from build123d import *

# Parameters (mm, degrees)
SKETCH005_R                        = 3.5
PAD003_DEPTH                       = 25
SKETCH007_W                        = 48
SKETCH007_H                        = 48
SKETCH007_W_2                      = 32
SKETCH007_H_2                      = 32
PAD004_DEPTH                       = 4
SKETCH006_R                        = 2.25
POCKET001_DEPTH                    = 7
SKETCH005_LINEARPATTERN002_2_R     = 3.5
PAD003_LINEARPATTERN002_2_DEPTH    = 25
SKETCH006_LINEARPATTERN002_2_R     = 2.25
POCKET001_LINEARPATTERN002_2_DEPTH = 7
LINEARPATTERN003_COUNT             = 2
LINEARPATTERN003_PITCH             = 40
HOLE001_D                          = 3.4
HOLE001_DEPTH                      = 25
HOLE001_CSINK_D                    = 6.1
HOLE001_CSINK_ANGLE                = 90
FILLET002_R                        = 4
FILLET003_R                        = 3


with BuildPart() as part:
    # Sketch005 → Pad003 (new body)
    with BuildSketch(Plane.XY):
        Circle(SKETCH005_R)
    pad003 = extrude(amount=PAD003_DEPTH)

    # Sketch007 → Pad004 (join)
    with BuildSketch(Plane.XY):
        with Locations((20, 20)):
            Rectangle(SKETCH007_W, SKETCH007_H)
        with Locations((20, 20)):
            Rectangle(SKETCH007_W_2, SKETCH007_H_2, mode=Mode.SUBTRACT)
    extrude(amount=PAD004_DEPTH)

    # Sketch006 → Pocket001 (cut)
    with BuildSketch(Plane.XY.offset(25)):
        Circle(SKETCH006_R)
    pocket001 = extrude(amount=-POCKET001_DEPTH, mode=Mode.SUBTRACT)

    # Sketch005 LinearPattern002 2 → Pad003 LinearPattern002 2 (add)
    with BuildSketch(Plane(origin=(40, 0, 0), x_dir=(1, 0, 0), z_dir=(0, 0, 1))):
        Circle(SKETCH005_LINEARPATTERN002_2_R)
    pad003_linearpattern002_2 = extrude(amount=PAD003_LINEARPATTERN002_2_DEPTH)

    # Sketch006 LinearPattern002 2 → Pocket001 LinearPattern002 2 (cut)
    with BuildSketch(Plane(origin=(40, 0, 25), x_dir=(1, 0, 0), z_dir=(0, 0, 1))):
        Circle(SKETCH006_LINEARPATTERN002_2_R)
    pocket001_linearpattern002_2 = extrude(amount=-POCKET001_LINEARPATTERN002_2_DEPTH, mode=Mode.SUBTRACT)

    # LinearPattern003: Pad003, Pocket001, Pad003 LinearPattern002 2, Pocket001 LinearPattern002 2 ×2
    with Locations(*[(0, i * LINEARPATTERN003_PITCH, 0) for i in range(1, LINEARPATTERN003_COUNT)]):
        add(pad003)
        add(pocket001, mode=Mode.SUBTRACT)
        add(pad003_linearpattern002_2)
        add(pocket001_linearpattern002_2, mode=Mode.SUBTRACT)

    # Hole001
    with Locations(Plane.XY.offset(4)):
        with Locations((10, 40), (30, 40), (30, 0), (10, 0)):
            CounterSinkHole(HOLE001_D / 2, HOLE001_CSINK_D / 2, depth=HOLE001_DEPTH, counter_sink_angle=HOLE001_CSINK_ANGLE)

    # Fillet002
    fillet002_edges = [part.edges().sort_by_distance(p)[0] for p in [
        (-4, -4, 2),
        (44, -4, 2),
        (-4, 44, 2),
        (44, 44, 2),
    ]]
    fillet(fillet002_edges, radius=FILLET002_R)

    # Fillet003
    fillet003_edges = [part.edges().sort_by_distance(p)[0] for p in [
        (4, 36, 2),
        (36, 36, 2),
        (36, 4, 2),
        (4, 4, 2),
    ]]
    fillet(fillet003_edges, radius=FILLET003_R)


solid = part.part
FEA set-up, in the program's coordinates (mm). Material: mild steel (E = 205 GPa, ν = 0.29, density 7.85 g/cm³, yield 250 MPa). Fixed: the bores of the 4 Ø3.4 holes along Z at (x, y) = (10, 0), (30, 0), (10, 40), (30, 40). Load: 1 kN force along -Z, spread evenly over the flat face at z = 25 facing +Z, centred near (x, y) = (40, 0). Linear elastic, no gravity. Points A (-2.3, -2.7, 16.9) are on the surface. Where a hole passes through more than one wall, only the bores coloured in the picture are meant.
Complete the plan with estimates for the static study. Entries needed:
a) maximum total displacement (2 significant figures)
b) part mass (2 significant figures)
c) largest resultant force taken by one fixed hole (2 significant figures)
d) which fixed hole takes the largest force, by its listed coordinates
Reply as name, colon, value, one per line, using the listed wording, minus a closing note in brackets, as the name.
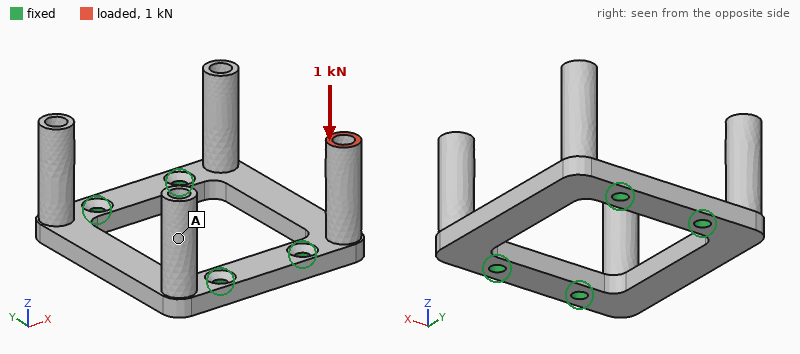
maximum total displacement: 0.13 mm
part mass: 60 g
largest resultant force taken by one fixed hole: 1.0 kN
which fixed hole takes the largest force, by its listed coordinates: (30, 0)
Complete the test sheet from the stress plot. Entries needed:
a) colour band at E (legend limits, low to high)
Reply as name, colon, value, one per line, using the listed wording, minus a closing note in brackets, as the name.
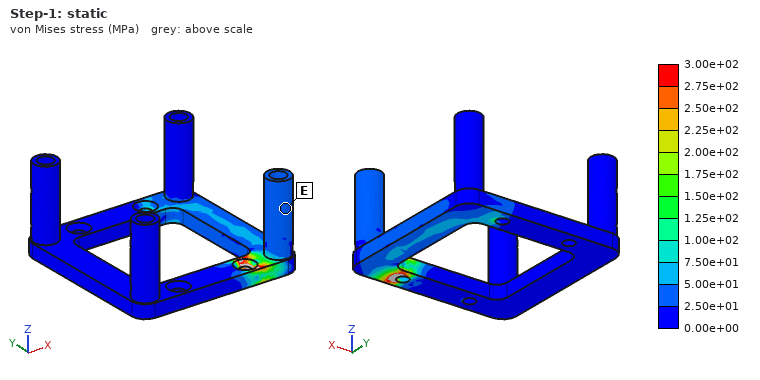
colour band at E: 2.50e+01 to 5.00e+01 MPa
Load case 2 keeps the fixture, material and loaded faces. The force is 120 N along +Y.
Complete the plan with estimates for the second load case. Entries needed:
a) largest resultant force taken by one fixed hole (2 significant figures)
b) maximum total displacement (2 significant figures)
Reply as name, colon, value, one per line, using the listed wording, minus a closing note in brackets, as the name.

largest resultant force taken by one fixed hole: 81 N
maximum total displacement: 52 µm
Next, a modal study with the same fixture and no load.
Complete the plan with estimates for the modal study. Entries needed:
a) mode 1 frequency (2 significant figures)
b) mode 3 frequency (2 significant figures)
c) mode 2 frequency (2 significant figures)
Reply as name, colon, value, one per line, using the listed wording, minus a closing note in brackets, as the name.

mode 1 frequency: 4000 Hz
mode 3 frequency: 5000 Hz
mode 2 frequency: 4000 Hz
